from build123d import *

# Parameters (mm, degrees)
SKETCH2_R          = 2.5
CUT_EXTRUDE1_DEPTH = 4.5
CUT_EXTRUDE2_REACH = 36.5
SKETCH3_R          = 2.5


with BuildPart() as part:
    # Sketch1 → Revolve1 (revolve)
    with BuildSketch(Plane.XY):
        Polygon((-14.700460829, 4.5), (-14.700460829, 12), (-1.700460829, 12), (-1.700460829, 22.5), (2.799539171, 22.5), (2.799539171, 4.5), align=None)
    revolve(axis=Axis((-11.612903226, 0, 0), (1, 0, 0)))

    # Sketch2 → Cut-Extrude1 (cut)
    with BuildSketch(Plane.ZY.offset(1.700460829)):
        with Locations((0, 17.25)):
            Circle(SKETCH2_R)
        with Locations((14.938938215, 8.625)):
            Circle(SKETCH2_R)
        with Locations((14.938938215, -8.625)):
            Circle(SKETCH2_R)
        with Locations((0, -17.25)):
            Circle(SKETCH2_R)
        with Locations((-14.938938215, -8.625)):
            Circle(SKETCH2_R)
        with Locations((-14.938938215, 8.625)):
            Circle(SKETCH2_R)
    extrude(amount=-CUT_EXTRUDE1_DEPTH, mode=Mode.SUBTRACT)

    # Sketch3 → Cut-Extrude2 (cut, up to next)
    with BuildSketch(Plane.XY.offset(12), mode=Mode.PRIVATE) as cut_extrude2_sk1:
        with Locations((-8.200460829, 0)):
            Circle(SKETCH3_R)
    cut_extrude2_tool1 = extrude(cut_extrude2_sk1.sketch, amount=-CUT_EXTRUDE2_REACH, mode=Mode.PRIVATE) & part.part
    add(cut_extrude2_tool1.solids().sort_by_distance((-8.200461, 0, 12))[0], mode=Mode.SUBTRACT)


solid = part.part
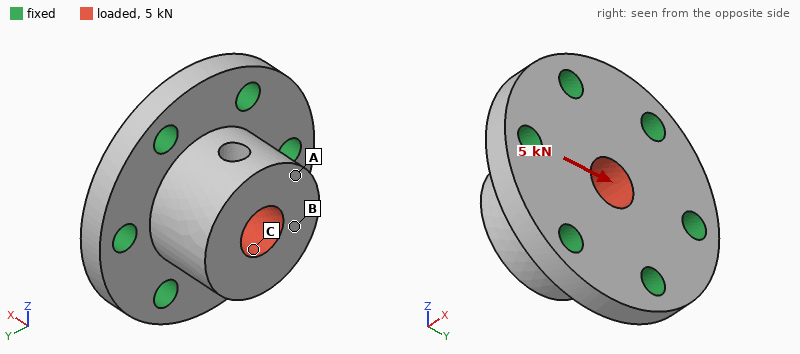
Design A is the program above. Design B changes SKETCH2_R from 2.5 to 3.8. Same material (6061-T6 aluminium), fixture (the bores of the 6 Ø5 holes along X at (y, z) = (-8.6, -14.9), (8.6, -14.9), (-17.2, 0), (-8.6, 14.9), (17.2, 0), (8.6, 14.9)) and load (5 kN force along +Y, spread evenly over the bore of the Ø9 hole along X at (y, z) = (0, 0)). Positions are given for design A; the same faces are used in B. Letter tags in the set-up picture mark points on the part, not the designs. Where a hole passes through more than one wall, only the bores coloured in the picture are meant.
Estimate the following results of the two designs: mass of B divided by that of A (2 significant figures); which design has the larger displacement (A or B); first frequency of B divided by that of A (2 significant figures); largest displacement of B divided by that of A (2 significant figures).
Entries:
0.94
A
1.1
0.81
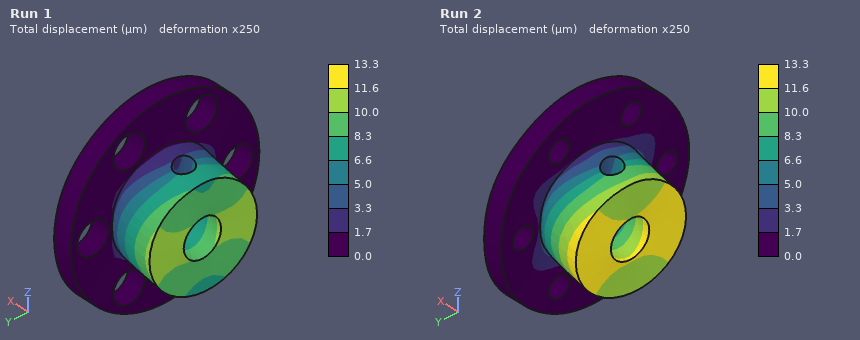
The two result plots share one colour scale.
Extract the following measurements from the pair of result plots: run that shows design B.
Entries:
Run 1
